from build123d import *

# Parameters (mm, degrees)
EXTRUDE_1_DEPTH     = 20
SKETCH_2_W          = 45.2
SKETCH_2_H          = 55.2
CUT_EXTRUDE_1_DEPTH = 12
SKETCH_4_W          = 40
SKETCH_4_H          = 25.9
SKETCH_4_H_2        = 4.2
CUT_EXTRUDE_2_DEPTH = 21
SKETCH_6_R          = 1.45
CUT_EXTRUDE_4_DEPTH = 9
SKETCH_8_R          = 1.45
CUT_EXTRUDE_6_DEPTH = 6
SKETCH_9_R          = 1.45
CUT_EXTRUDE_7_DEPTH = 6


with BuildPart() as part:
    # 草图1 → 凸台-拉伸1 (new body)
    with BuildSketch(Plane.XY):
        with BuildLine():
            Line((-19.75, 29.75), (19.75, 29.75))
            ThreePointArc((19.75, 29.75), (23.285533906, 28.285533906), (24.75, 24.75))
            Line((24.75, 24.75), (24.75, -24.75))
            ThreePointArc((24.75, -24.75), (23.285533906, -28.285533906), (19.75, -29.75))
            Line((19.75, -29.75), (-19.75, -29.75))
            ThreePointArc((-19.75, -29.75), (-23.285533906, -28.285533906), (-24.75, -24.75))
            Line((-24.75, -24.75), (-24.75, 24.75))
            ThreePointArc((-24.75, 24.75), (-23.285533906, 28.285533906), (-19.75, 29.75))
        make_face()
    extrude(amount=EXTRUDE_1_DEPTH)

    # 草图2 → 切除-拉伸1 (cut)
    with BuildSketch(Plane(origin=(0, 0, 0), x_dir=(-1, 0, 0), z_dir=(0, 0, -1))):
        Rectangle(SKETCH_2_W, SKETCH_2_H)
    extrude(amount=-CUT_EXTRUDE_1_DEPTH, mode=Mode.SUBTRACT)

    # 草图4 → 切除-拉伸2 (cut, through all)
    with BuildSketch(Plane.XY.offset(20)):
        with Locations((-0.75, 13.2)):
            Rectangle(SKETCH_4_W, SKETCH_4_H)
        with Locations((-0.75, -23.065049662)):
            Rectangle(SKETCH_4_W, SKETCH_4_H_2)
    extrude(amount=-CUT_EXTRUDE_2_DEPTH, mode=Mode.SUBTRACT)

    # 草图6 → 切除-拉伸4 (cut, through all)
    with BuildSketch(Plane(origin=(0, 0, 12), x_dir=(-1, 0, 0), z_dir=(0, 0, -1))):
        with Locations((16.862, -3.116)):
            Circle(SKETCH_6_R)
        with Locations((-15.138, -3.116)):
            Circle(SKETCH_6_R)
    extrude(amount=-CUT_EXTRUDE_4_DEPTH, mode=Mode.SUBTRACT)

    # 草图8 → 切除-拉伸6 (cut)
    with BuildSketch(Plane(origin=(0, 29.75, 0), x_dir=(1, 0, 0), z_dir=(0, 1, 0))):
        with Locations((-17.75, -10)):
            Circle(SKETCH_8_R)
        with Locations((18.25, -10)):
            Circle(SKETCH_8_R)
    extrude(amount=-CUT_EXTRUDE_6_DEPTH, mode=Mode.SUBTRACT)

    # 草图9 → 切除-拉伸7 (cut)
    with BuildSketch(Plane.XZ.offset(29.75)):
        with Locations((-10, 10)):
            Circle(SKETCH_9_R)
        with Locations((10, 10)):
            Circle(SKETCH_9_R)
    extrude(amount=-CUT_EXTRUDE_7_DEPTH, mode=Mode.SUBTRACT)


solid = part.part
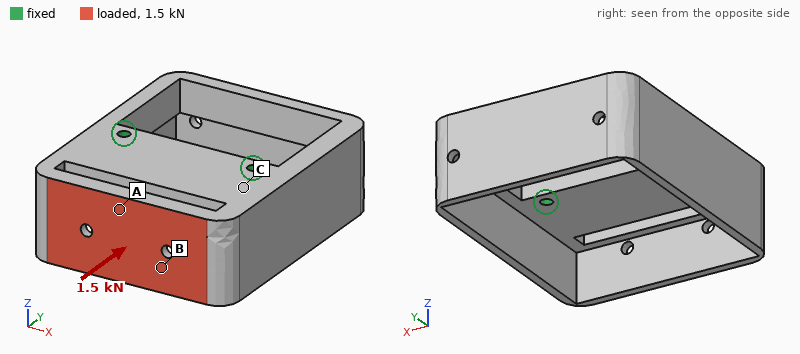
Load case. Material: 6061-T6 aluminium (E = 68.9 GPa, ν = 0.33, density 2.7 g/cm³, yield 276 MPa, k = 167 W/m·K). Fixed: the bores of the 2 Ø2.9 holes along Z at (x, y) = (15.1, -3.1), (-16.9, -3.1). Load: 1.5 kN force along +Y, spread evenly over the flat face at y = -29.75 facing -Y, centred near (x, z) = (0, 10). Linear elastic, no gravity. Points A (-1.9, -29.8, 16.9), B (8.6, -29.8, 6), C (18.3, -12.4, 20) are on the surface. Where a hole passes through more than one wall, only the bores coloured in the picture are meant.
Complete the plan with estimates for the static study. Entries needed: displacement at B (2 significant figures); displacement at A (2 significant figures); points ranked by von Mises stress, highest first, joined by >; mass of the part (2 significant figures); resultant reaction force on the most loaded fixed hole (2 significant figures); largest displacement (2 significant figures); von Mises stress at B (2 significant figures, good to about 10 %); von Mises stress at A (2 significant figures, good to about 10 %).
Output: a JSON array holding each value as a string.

["0.19 mm", "0.11 mm", "A > B > C", "51 g", "850 N", "0.32 mm", "83 MPa", "120 MPa"]
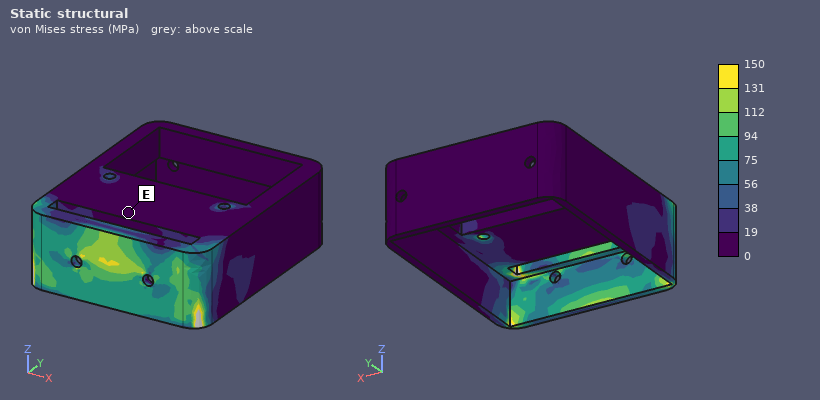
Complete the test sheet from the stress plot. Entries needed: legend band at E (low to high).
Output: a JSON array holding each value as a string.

["0 to 19 MPa"]
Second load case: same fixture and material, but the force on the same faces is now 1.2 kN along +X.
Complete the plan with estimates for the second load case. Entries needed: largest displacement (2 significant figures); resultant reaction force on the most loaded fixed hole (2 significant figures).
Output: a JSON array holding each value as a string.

["49 µm", "1.1 kN"]
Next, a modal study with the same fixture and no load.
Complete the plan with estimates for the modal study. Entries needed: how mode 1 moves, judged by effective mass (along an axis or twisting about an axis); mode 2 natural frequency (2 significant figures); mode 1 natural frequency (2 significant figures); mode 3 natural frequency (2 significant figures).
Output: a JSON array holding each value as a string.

["along X", "3400 Hz", "2500 Hz", "5200 Hz"]
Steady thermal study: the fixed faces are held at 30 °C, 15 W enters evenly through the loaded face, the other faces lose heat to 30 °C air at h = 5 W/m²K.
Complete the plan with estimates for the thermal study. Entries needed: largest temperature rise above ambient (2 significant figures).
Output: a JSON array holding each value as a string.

["23 K"]
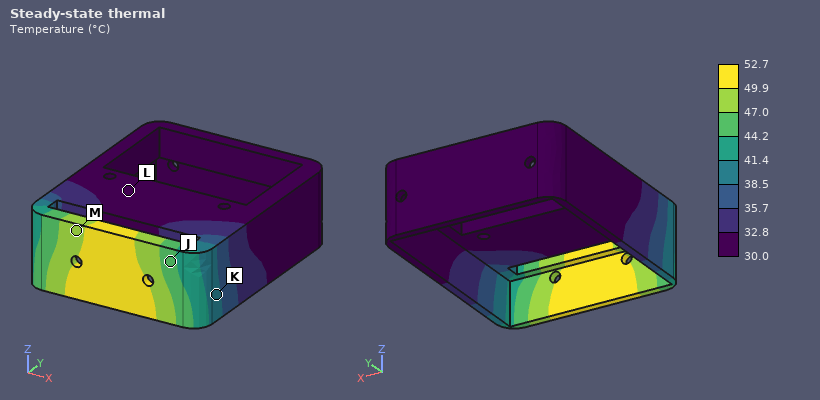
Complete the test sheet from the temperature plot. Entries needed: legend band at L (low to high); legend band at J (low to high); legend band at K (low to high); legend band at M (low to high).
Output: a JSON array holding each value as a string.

["30.0 to 32.8 °C", "44.2 to 47.0 °C", "38.5 to 41.4 °C", "47.0 to 49.9 °C"]
